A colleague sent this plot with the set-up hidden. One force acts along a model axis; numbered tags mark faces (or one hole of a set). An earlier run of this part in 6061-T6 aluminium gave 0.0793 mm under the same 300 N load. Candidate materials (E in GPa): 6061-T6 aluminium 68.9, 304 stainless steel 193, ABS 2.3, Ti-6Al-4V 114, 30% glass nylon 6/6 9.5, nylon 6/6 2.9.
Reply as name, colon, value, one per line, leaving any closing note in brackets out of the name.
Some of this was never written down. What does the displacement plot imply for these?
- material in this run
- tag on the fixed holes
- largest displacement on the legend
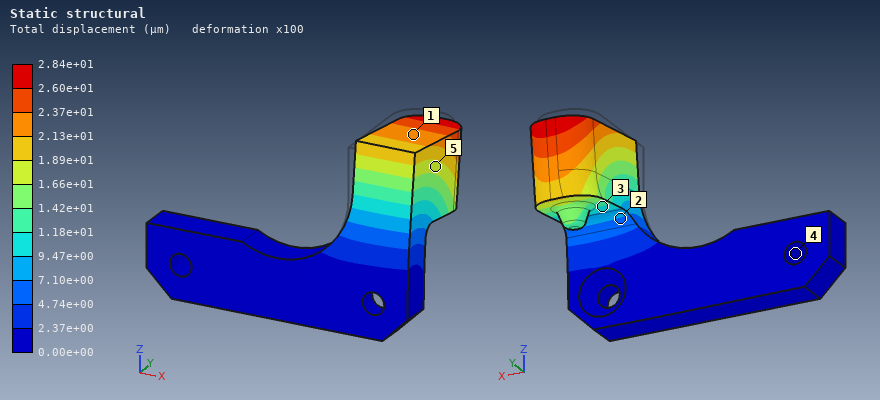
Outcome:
material in this run: 304 stainless steel
tag on the fixed holes: 4
largest displacement on the legend: 2.84e+01 µm
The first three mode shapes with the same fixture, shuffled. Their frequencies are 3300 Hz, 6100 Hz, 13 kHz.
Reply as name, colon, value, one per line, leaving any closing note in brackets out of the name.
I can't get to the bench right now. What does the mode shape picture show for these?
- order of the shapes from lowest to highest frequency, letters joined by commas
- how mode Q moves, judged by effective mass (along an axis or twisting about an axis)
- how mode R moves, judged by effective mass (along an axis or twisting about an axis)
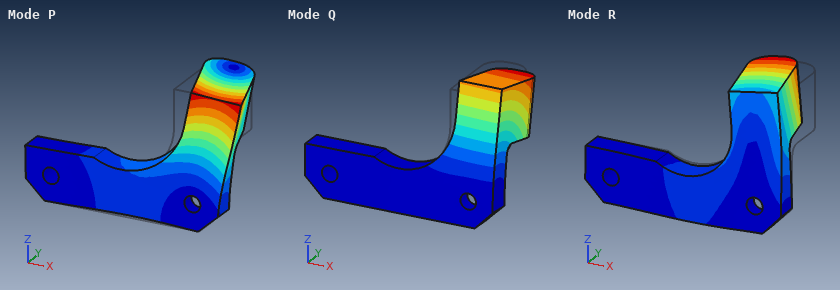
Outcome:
order of the shapes from lowest to highest frequency, letters joined by commas: Q, R, P
how mode Q moves, judged by effective mass: along Y
how mode R moves, judged by effective mass: along X
